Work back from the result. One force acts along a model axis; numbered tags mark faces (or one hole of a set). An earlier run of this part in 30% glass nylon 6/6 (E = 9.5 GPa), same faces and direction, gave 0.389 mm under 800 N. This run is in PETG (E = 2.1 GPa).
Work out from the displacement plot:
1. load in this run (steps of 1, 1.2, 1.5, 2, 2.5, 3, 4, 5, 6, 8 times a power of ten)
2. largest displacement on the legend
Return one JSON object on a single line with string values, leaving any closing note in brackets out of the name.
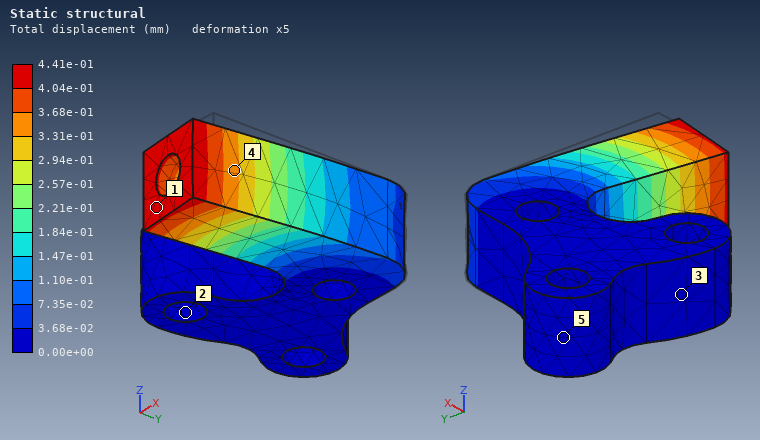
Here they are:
{"load in this run": "200 N", "largest displacement on the legend": "4.41e-01 mm"}
